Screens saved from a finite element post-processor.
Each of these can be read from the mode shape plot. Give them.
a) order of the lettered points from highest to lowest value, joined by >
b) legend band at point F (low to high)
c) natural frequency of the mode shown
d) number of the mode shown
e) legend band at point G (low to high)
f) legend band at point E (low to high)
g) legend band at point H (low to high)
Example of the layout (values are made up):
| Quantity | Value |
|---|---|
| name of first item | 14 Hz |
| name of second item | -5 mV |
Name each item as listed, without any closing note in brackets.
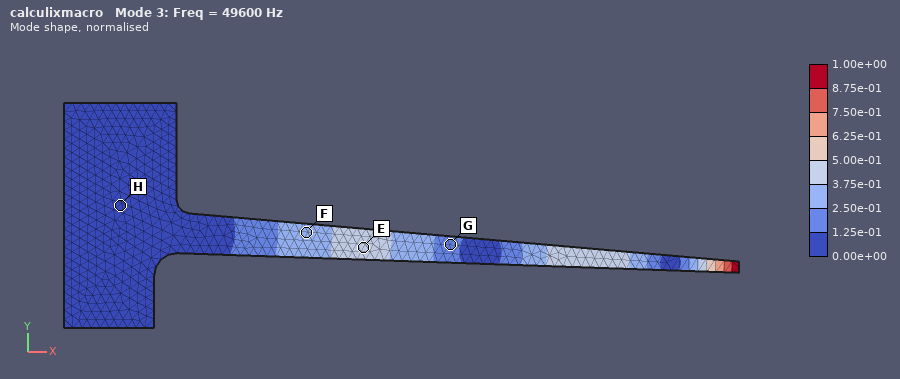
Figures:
| Quantity | Value |
|---|---|
| order of the lettered points from highest to lowest value, joined by > | E > F > G > H |
| legend band at point F | 2.50e-01 to 3.75e-01 |
| natural frequency of the mode shown | 49600 Hz |
| number of the mode shown | 3 |
| legend band at point G | 1.25e-01 to 2.50e-01 |
| legend band at point E | 3.75e-01 to 5.00e-01 |
| legend band at point H | 0.00e+00 to 1.25e-01 |
